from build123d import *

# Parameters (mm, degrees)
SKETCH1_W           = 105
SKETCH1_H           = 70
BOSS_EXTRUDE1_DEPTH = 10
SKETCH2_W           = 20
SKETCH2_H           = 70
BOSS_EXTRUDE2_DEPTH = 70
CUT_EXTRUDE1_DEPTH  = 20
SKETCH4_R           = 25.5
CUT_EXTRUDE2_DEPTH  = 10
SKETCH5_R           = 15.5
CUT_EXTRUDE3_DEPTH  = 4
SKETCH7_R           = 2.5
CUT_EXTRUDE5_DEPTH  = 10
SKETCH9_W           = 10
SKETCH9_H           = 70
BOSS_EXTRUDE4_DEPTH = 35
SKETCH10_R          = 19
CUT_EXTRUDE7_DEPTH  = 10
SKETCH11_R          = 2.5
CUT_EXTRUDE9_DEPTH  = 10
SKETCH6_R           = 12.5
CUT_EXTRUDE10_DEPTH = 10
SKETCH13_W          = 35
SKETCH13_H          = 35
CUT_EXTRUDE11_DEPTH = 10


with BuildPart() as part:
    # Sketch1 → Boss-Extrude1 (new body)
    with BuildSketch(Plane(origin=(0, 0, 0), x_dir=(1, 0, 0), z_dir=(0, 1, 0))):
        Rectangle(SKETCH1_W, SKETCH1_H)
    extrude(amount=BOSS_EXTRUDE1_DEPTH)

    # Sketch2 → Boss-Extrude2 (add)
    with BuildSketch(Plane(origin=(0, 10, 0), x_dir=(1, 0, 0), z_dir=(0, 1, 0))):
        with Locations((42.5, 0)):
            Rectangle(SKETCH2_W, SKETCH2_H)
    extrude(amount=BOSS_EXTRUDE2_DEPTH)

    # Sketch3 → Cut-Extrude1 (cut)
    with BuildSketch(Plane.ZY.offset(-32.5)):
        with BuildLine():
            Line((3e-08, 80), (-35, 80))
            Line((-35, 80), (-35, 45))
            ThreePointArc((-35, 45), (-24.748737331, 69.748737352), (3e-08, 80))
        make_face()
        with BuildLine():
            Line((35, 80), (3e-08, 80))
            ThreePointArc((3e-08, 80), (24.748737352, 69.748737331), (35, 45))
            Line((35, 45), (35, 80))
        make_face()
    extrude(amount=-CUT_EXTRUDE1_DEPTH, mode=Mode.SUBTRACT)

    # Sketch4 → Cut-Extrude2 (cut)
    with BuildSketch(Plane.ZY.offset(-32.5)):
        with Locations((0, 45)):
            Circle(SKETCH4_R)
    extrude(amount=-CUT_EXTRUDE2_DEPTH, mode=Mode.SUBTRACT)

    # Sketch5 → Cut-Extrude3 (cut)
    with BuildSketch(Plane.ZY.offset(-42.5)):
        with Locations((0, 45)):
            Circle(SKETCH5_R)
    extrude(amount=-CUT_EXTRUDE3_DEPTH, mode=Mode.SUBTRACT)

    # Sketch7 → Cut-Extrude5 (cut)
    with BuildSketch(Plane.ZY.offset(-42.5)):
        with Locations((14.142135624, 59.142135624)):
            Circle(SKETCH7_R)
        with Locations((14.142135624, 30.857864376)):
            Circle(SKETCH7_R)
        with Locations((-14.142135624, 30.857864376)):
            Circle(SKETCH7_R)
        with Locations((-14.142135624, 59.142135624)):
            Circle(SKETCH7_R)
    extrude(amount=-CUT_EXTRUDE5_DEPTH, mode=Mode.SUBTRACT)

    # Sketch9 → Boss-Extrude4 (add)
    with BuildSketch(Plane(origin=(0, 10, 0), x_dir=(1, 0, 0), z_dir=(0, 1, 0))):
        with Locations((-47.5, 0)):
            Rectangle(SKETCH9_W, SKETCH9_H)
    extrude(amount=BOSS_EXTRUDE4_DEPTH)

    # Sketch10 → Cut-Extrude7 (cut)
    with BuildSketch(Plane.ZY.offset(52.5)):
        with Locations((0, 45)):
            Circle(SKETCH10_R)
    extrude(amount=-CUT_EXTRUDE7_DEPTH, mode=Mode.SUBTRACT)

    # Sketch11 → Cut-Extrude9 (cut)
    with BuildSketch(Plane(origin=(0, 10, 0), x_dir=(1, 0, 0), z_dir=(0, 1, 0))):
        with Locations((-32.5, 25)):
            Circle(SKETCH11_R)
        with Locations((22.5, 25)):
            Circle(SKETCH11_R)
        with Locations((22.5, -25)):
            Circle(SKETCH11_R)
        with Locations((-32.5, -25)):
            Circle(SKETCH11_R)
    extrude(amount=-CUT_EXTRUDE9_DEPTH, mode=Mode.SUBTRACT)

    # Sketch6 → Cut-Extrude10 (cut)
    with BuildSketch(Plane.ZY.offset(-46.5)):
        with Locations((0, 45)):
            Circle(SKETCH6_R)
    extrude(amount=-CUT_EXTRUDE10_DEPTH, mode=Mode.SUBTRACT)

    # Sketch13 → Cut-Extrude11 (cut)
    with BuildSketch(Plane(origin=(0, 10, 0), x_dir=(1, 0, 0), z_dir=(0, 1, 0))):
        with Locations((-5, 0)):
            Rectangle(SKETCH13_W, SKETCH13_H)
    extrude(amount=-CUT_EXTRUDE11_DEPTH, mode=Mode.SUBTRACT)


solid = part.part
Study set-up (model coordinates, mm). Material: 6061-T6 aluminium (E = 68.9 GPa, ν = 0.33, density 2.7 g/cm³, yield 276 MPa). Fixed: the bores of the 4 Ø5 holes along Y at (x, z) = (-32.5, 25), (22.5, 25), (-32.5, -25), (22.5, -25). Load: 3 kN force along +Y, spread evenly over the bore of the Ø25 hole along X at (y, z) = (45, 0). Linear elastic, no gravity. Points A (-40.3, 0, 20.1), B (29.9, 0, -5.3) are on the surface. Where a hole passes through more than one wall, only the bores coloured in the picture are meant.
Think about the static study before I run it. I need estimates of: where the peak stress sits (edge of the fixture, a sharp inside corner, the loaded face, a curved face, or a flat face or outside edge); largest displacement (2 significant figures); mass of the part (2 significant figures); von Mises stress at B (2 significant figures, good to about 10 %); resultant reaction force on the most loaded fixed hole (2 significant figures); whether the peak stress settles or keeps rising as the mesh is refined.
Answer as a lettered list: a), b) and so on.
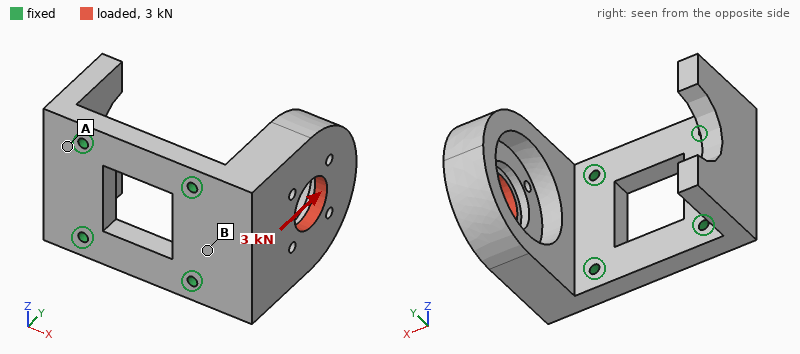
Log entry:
a) edge of the fixture
b) 0.25 mm
c) 380 g
d) 26 MPa
e) 1.6 kN
f) keeps rising
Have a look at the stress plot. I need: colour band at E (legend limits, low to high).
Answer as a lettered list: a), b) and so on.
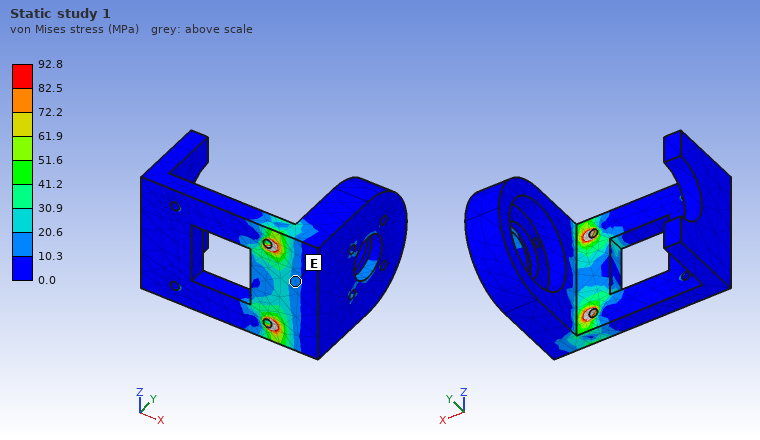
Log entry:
a) 10.3 to 20.6 MPa
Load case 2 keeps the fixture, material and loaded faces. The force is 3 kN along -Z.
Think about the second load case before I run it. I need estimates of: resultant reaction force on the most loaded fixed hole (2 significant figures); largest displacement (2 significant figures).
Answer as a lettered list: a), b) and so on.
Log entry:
a) 3.1 kN
b) 68 µm
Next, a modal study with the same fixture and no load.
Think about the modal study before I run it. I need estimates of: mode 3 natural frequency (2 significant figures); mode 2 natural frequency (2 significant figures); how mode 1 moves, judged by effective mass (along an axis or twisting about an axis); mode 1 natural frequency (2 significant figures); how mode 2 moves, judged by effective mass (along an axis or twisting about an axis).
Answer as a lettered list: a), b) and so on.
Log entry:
a) 3800 Hz
b) 3000 Hz
c) along X
d) 1200 Hz
e) along Z
